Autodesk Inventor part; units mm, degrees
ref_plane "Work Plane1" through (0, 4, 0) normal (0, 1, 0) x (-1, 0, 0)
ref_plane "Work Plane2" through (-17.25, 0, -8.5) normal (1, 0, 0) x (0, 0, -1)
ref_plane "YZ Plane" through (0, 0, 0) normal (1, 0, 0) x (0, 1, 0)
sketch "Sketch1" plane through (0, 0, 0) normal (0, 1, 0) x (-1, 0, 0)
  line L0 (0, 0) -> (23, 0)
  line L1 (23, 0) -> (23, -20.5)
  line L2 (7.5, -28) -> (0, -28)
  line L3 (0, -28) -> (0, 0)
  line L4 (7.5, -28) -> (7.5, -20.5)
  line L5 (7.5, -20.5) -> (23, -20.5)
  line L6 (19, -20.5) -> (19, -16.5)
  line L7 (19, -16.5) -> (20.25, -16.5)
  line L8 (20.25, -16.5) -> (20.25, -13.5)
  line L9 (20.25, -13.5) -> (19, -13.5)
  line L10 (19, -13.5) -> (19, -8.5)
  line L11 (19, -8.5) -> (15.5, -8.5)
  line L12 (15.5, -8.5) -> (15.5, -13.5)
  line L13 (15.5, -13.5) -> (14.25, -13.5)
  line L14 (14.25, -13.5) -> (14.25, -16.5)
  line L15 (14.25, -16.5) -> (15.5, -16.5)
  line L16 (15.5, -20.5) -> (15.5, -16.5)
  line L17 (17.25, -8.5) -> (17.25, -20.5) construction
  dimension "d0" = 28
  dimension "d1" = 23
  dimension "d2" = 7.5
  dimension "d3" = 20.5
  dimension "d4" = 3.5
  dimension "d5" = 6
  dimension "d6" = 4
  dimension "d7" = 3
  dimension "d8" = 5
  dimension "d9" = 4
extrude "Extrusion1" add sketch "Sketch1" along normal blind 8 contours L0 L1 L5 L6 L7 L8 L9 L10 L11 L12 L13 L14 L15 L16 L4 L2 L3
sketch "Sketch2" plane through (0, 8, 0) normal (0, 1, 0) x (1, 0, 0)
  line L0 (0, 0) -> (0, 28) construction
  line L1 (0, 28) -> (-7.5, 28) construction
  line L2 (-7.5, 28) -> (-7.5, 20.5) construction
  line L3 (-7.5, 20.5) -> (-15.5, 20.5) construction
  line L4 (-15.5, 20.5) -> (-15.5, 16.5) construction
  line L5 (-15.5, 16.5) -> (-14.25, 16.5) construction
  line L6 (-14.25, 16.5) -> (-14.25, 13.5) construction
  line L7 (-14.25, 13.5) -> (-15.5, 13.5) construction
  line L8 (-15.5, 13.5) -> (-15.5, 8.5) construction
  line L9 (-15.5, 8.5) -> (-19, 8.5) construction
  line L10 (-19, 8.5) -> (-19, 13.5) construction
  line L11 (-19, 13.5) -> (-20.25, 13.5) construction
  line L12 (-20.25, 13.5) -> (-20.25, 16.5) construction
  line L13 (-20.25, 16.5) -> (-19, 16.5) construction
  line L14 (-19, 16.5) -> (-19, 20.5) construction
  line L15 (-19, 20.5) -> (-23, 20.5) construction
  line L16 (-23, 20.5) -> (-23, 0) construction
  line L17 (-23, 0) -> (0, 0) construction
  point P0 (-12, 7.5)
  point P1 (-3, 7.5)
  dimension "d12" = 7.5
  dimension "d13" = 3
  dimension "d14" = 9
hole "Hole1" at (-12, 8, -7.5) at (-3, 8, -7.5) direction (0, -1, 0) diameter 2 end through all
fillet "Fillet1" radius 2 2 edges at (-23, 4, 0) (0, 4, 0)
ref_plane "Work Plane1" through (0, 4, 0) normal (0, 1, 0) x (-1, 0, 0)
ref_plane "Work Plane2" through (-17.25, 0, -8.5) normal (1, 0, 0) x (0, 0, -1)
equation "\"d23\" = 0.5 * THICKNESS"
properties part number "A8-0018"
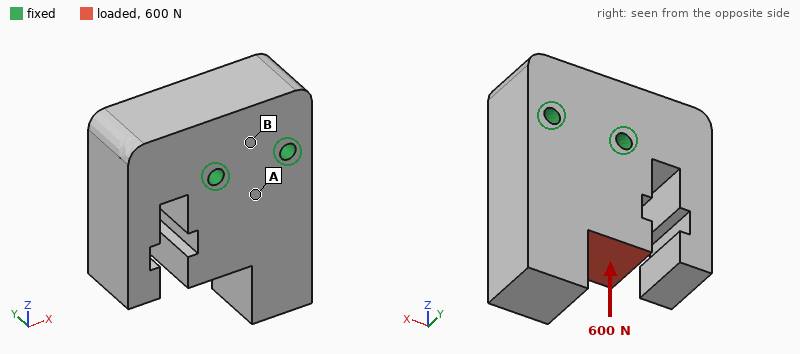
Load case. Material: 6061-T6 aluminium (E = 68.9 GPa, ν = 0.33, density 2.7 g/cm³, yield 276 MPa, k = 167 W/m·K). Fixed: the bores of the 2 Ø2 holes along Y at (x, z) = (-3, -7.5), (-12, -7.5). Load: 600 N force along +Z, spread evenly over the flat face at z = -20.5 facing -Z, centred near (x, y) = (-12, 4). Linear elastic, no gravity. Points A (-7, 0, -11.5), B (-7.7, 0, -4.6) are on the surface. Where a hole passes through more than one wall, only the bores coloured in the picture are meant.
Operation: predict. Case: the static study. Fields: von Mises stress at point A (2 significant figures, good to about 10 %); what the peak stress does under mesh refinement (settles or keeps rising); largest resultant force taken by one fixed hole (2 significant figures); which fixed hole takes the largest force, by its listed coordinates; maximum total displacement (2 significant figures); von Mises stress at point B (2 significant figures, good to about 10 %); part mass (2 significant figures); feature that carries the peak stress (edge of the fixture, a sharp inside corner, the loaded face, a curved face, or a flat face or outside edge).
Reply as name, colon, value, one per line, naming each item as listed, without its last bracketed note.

von Mises stress at point A: 3.1 MPa
what the peak stress does under mesh refinement: keeps rising
largest resultant force taken by one fixed hole: 550 N
which fixed hole takes the largest force, by its listed coordinates: (-12, -7.5)
maximum total displacement: 3.5 µm
von Mises stress at point B: 1.7 MPa
part mass: 10 g
feature that carries the peak stress: edge of the fixture
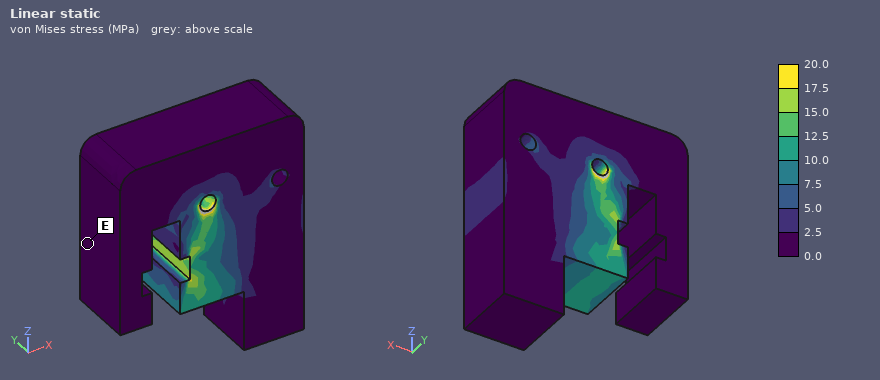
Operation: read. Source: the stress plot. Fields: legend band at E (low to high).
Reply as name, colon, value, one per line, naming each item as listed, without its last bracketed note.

legend band at E: 0.0 to 2.5 MPa
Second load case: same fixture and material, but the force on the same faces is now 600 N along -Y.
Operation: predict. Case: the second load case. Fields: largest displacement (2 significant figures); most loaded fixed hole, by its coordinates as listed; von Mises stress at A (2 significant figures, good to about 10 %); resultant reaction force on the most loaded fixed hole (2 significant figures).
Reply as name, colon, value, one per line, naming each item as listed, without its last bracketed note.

largest displacement: 21 µm
most loaded fixed hole, by its coordinates as listed: (-12, -7.5)
von Mises stress at A: 30 MPa
resultant reaction force on the most loaded fixed hole: 470 N
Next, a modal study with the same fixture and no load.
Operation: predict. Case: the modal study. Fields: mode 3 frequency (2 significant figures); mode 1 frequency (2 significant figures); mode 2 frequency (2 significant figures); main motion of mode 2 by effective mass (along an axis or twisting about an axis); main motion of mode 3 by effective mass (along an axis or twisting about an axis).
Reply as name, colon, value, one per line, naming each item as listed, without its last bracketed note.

mode 3 frequency: 17 kHz
mode 1 frequency: 13 kHz
mode 2 frequency: 16 kHz
main motion of mode 2 by effective mass: along Y
main motion of mode 3 by effective mass: along Y
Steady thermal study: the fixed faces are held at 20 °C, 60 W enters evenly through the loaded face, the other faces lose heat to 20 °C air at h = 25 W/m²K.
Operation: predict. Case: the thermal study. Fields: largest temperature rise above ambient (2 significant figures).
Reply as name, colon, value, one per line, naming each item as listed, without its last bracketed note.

largest temperature rise above ambient: 57 K
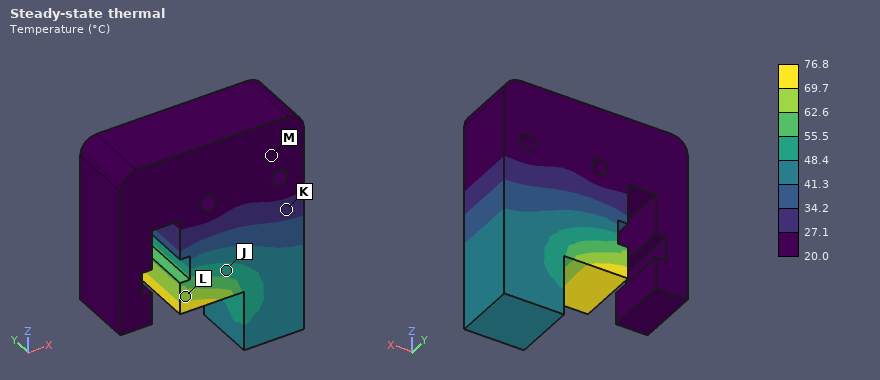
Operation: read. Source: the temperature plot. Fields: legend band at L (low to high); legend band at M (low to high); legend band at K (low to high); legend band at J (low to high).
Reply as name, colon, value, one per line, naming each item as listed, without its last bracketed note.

legend band at L: 62.6 to 69.7 °C
legend band at M: 20.0 to 27.1 °C
legend band at K: 27.1 to 34.2 °C
legend band at J: 48.4 to 55.5 °C
